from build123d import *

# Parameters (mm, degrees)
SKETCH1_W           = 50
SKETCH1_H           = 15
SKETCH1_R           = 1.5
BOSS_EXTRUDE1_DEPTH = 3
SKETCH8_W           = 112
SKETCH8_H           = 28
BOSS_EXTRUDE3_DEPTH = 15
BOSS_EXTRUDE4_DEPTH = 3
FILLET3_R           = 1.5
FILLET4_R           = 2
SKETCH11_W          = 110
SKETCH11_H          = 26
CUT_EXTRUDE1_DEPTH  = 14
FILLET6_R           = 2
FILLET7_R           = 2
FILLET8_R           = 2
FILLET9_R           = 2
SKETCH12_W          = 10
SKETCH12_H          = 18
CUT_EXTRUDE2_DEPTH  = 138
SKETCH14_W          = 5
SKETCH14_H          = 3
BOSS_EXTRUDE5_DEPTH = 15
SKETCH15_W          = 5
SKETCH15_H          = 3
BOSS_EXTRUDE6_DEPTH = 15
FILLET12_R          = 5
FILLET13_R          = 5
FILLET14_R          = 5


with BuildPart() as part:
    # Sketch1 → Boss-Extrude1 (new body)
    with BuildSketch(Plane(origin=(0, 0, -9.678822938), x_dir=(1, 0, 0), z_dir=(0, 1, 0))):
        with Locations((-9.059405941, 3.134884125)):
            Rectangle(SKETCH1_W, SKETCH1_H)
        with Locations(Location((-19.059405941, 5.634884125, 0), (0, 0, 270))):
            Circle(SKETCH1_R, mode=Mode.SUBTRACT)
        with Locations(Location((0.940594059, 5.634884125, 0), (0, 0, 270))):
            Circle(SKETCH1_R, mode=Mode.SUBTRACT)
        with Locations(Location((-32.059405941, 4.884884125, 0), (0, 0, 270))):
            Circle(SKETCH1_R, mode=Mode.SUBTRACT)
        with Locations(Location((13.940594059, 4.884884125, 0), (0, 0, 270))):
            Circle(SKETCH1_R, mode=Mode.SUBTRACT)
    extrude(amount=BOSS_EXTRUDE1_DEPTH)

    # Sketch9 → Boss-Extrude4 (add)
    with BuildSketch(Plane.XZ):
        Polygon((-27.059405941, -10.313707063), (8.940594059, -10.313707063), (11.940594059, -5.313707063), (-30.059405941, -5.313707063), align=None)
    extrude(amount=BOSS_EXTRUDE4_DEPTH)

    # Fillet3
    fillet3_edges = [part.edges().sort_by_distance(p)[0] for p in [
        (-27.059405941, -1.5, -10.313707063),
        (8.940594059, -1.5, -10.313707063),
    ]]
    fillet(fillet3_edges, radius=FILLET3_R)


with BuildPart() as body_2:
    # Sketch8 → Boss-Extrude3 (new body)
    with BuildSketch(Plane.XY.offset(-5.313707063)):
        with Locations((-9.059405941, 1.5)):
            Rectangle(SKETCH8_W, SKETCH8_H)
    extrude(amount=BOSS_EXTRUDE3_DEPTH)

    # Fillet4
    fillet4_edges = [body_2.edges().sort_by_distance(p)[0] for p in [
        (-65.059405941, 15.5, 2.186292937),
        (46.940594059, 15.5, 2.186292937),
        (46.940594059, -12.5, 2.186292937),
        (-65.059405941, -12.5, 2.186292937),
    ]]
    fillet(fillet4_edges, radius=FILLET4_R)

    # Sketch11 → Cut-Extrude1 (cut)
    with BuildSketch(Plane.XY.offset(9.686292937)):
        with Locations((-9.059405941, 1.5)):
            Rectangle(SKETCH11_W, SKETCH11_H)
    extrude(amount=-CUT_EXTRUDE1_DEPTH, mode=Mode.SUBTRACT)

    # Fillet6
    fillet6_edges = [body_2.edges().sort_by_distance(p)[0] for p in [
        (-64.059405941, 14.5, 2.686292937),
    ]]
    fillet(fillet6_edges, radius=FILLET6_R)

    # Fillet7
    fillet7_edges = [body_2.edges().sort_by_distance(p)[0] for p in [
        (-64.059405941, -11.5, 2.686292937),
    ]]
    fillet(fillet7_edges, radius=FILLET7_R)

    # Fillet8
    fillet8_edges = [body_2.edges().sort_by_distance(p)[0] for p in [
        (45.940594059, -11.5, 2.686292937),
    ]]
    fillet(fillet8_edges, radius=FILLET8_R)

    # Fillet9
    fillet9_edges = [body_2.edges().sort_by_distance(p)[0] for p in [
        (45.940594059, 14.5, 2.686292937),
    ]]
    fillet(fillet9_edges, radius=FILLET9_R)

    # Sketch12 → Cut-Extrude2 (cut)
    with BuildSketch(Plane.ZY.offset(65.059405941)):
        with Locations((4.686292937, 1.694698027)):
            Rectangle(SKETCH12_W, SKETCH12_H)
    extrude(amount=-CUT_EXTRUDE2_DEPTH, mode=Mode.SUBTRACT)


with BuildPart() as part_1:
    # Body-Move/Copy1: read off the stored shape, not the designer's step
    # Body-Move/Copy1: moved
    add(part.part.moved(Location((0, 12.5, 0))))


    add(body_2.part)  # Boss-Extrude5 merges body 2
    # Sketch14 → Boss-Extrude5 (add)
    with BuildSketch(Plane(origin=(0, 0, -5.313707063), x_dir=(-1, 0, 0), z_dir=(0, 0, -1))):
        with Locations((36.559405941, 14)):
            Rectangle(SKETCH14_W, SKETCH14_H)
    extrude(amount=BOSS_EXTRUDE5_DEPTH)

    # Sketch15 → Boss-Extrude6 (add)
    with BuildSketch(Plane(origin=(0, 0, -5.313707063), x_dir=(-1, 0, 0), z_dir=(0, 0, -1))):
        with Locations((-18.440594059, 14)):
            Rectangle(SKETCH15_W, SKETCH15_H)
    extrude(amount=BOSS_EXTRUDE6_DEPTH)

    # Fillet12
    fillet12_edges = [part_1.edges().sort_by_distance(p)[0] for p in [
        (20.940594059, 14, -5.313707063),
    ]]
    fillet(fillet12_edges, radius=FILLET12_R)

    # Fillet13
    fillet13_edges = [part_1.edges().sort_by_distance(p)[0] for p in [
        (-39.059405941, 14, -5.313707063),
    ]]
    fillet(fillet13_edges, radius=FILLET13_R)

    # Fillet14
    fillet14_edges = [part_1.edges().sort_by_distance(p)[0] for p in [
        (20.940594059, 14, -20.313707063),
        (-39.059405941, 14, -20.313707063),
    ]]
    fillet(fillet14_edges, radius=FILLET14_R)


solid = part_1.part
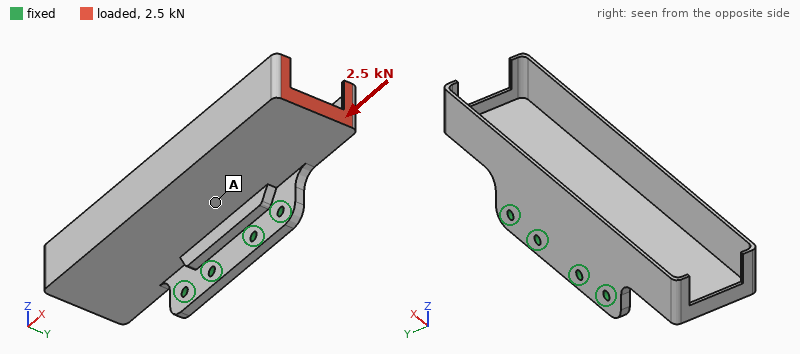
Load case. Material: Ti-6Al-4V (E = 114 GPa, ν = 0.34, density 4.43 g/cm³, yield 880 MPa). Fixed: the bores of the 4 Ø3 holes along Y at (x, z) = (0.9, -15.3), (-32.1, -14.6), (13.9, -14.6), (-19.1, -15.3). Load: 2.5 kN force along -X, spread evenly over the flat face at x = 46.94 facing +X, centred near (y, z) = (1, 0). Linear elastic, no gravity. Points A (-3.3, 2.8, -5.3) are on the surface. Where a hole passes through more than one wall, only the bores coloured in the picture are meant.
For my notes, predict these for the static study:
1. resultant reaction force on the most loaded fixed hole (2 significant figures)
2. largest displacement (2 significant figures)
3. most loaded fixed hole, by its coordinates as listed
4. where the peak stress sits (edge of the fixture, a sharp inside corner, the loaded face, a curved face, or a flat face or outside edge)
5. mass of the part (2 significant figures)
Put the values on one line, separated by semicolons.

1.2 kN; 1.2 mm; (13.9, -14.6); the loaded face; 44 g
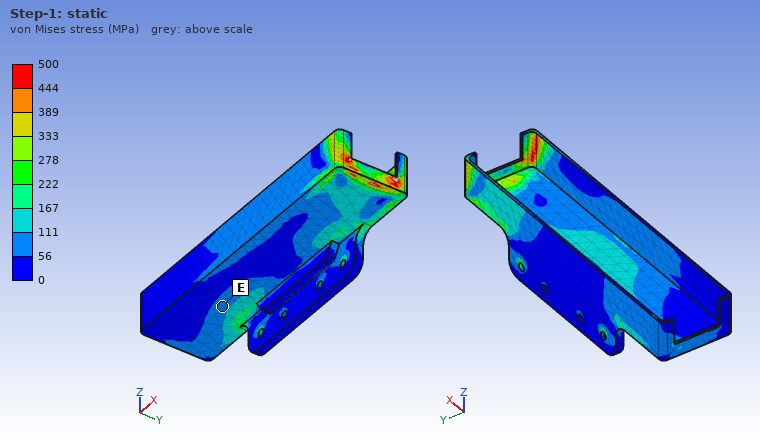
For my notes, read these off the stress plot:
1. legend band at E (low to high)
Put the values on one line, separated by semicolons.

56 to 111 MPa
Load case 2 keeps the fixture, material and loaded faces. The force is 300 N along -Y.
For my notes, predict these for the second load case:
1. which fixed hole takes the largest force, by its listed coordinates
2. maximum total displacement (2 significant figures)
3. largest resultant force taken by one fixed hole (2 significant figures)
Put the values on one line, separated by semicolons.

(13.9, -14.6); 1.1 mm; 470 N
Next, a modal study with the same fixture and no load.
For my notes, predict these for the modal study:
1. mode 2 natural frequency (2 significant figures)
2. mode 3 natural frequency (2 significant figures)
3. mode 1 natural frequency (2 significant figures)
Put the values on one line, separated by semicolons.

690 Hz; 2900 Hz; 680 Hz
